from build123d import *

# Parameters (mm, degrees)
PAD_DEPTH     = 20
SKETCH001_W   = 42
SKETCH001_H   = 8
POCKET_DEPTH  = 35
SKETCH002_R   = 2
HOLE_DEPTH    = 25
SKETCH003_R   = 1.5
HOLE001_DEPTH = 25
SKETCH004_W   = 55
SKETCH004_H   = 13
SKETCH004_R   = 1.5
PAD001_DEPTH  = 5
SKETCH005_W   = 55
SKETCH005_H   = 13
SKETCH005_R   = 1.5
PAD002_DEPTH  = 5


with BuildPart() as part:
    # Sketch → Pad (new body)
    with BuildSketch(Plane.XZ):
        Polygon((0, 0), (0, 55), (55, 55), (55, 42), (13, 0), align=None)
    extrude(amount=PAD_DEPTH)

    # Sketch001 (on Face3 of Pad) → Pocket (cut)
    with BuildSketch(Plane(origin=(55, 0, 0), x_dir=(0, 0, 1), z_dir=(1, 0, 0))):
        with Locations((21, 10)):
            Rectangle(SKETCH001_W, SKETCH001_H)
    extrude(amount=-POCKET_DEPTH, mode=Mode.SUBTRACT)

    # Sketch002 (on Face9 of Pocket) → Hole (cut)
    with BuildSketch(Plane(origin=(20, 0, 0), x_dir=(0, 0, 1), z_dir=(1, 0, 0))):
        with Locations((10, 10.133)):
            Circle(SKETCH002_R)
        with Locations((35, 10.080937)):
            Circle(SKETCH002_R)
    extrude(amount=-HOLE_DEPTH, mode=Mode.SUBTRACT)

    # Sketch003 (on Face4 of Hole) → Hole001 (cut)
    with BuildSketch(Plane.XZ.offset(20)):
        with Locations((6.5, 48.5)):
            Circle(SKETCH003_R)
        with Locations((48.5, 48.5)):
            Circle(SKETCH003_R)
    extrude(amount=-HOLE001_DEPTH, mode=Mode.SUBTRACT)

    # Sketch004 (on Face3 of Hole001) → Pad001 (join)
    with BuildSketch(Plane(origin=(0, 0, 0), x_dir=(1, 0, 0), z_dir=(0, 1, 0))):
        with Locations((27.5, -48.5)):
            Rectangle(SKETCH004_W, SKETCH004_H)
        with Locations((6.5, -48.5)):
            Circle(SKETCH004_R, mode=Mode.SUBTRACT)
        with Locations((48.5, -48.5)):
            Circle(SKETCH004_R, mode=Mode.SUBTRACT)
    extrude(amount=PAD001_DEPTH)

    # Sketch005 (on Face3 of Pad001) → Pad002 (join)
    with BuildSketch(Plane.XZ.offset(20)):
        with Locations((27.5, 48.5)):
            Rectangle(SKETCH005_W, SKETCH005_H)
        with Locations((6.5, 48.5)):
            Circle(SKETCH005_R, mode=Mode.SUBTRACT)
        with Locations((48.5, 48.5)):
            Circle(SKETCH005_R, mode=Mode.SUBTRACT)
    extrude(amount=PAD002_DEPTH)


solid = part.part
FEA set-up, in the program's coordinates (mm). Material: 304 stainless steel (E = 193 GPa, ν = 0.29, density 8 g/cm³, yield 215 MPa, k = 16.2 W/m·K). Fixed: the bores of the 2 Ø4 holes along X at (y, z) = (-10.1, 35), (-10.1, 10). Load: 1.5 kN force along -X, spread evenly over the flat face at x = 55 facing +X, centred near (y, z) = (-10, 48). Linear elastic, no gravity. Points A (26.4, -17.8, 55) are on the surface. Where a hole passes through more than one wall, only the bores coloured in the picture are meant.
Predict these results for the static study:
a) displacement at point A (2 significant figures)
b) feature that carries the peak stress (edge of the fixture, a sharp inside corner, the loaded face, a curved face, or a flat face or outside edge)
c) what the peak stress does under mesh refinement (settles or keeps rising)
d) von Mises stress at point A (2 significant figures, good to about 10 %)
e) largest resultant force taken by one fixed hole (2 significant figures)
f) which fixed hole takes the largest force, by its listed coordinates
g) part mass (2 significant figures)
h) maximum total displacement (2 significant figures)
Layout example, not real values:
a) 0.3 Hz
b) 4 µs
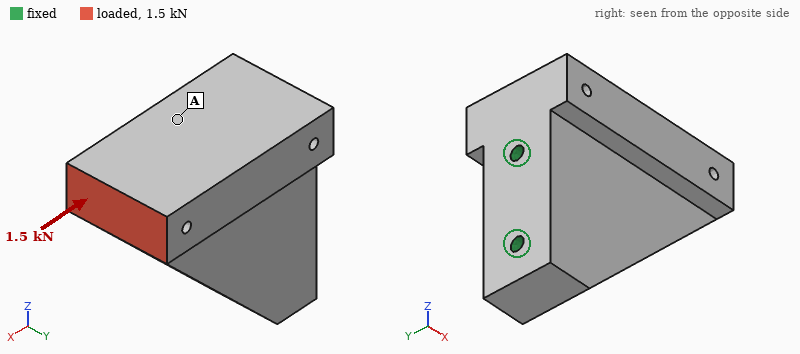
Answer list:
a) 1.6 µm
b) edge of the fixture
c) keeps rising
d) 3.7 MPa
e) 1.8 kN
f) (-10.1, 35)
g) 350 g
h) 3.1 µm
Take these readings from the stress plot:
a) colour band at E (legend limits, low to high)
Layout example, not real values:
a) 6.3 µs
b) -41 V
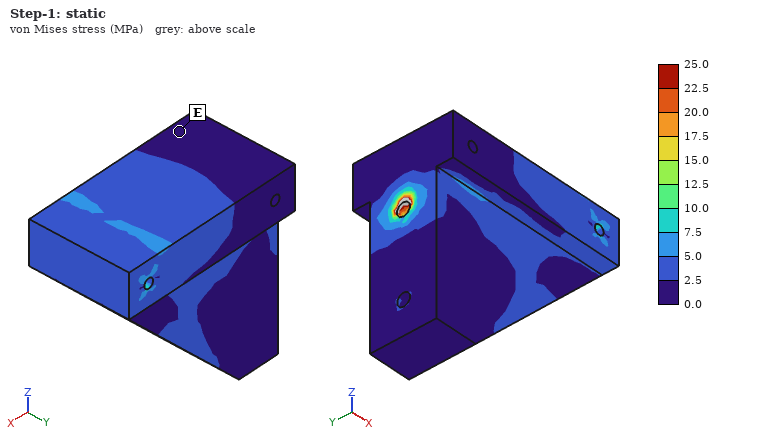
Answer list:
a) 0.0 to 2.5 MPa
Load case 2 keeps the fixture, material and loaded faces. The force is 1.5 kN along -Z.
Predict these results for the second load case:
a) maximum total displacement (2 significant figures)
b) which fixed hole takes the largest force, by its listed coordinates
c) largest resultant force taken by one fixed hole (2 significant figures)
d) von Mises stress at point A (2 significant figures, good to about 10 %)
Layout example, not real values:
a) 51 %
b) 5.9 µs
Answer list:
a) 8.9 µm
b) (-10.1, 10)
c) 1.9 kN
d) 8.8 MPa
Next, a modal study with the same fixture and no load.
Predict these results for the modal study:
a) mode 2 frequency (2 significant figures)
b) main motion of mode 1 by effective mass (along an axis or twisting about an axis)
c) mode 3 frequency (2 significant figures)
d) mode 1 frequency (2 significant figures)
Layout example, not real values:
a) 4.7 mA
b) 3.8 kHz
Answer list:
a) 9000 Hz
b) along Y
c) 11 kHz
d) 5600 Hz
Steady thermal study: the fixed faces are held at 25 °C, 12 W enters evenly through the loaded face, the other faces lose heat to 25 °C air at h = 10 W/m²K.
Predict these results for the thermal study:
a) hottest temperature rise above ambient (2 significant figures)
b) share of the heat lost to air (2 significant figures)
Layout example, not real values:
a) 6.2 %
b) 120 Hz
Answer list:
a) 63 K
b) 16 %
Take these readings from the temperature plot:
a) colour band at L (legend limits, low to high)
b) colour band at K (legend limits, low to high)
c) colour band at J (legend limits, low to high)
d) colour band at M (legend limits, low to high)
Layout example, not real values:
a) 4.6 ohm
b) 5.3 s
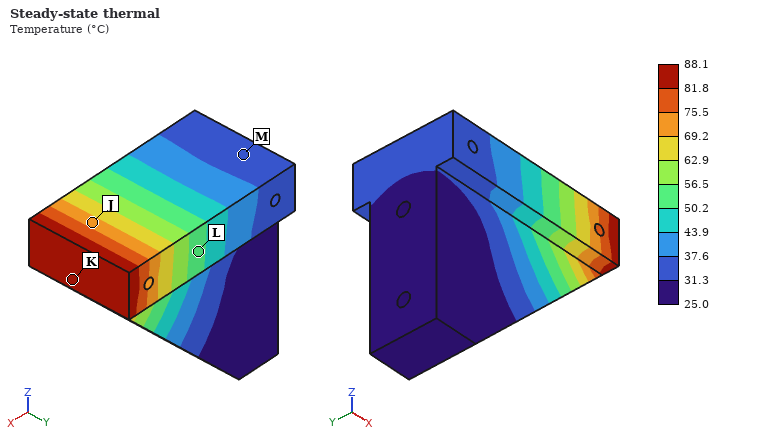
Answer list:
a) 50.2 to 56.5 °C
b) 81.8 to 88.1 °C
c) 69.2 to 75.5 °C
d) 31.3 to 37.6 °C
